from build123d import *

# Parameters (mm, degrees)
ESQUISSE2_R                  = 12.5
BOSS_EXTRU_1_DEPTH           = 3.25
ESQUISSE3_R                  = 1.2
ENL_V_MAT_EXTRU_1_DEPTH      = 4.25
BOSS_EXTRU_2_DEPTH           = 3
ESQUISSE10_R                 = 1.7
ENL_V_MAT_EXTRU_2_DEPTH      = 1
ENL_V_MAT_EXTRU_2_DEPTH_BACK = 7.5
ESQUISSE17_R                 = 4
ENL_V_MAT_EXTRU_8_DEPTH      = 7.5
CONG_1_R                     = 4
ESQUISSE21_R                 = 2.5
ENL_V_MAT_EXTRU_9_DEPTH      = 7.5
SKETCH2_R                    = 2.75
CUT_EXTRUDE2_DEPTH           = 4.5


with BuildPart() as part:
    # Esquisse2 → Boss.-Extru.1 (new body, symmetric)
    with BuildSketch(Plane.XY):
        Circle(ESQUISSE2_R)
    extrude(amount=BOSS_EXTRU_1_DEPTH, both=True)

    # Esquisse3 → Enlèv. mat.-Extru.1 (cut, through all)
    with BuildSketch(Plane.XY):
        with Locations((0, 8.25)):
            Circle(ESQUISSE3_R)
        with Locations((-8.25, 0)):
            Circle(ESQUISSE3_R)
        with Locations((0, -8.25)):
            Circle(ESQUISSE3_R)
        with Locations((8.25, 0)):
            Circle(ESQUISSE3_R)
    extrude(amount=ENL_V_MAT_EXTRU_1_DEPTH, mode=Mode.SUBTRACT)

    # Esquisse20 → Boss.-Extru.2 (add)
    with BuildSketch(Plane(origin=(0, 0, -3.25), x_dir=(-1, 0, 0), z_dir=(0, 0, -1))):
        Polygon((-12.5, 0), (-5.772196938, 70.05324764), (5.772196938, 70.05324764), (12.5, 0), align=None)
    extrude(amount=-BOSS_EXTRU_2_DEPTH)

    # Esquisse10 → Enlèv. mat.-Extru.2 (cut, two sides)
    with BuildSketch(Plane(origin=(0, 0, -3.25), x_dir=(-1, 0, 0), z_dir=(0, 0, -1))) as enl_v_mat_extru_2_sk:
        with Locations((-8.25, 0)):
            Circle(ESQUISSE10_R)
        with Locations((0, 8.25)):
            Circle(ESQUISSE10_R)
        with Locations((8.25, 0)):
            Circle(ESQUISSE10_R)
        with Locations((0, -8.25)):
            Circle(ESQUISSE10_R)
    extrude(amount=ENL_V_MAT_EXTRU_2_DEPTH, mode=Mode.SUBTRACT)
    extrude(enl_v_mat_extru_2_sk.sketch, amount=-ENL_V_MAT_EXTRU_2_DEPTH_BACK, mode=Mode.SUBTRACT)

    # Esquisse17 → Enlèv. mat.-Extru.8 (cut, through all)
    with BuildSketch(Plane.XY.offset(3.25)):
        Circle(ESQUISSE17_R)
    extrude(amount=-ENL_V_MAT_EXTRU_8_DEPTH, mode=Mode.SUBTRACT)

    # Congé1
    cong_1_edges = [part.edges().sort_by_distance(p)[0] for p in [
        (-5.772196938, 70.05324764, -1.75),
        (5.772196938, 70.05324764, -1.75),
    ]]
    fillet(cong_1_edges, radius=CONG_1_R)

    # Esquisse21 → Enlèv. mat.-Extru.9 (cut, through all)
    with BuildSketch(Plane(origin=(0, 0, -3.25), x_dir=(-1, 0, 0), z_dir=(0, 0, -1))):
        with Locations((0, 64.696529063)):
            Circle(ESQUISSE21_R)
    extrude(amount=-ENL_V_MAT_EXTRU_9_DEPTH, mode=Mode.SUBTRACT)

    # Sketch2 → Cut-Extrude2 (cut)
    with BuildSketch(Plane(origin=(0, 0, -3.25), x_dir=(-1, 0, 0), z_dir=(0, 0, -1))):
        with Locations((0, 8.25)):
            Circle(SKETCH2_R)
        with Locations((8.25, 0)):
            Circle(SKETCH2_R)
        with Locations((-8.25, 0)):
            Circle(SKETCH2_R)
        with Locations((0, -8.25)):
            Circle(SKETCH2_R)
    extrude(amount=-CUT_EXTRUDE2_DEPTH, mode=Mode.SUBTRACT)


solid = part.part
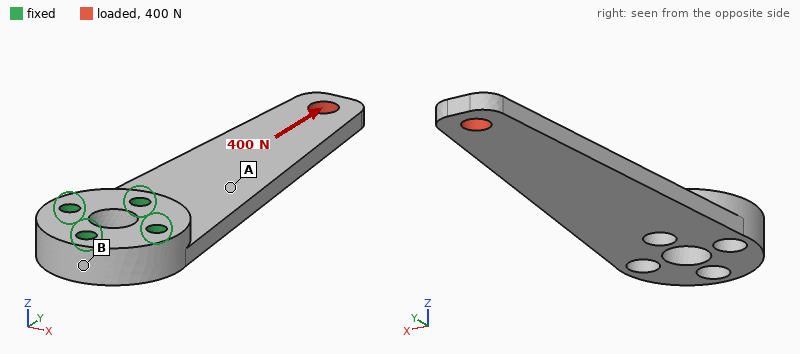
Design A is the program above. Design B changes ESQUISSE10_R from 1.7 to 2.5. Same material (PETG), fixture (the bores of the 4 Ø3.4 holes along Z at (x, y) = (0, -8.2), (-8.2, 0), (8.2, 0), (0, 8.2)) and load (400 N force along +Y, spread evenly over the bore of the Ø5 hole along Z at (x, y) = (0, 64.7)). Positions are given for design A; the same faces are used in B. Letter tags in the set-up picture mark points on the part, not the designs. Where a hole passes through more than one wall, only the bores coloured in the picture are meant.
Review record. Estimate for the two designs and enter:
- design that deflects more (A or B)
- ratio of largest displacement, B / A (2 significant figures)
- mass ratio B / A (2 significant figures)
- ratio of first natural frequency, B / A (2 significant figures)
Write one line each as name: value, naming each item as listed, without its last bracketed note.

design that deflects more: A
ratio of largest displacement, B / A: 0.83
mass ratio B / A: 0.98
ratio of first natural frequency, B / A: 1.0
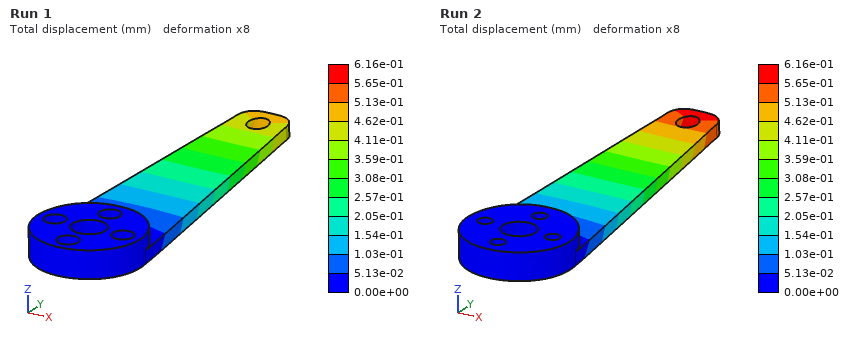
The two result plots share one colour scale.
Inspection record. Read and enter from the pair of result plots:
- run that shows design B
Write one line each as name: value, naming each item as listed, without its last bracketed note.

run that shows design B: Run 1
